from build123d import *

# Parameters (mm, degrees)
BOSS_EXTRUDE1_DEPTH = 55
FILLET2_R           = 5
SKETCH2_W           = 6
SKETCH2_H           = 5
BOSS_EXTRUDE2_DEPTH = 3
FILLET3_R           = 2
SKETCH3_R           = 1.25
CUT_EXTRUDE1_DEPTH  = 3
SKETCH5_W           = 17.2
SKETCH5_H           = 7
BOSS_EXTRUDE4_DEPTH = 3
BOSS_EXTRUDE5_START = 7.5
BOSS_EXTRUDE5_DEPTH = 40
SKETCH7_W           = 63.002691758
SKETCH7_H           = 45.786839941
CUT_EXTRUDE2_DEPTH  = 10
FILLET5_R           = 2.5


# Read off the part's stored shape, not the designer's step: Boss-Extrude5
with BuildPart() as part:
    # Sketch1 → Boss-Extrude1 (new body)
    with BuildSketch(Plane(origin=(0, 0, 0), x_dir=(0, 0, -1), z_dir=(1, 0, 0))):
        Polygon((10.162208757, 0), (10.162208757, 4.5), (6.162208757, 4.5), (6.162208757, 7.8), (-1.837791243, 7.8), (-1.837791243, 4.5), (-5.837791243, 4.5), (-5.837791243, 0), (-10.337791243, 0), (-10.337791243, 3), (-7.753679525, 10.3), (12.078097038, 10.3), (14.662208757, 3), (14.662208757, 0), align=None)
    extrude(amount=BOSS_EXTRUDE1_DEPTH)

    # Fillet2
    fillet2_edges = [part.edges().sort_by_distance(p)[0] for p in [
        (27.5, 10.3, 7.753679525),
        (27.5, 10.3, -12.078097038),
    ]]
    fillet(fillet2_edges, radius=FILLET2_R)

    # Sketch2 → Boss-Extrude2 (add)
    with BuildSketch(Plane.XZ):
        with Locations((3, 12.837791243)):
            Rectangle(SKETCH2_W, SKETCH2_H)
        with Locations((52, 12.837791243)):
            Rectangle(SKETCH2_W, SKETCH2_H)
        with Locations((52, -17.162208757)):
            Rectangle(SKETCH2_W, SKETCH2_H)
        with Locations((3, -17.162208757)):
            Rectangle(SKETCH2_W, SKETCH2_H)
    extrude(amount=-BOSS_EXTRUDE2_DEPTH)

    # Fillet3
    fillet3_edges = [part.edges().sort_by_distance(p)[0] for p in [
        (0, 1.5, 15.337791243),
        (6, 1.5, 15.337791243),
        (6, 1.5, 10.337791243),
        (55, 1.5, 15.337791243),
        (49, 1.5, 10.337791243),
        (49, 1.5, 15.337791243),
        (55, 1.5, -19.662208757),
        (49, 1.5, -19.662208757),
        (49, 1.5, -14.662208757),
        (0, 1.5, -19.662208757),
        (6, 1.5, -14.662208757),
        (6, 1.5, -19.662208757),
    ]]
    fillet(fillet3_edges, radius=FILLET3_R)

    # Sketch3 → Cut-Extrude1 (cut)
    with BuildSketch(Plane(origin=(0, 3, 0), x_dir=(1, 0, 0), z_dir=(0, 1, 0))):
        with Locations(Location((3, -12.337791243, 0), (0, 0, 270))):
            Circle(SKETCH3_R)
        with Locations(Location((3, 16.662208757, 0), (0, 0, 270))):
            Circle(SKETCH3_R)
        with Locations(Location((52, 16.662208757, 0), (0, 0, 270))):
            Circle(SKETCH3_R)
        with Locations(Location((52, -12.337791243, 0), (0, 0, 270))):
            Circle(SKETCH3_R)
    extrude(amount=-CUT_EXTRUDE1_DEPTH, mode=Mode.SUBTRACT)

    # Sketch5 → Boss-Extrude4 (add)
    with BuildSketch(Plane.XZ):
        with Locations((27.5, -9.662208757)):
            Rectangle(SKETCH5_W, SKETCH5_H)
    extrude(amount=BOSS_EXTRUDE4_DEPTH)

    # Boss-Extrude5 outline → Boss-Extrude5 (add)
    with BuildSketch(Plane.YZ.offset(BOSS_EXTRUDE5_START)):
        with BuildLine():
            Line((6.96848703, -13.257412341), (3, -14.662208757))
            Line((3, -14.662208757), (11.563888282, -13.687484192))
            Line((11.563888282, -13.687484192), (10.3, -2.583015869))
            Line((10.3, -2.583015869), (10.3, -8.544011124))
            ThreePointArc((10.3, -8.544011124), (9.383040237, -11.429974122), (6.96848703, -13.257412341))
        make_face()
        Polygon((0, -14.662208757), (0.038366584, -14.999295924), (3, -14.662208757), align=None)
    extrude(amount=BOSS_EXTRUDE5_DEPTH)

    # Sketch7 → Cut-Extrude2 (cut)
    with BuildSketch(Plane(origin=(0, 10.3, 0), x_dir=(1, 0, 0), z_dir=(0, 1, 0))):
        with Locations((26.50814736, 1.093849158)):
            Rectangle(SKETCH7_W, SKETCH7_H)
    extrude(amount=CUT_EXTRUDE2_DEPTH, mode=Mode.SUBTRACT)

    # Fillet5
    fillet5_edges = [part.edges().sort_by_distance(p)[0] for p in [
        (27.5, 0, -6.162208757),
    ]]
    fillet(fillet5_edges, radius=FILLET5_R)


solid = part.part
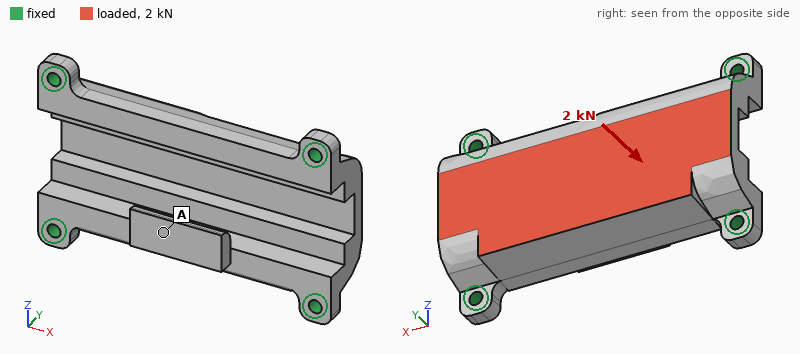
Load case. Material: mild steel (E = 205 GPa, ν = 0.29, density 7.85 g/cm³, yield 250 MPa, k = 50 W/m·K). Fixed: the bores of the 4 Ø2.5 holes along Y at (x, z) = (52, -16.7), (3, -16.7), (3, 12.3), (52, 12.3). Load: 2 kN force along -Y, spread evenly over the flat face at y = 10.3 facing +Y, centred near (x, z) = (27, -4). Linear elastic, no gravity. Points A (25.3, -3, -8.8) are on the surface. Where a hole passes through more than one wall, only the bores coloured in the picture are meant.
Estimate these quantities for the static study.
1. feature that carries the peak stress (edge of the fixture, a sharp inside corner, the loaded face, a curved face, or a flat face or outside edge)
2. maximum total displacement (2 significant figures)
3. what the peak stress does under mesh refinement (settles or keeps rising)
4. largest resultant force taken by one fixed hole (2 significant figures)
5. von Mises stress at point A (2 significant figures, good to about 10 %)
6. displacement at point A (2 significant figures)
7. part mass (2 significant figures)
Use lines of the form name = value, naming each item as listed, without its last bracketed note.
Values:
feature that carries the peak stress = edge of the fixture
maximum total displacement = 9.8 µm
what the peak stress does under mesh refinement = keeps rising
largest resultant force taken by one fixed hole = 850 N
von Mises stress at point A = 10.0 MPa
displacement at point A = 9.0 µm
part mass = 66 g
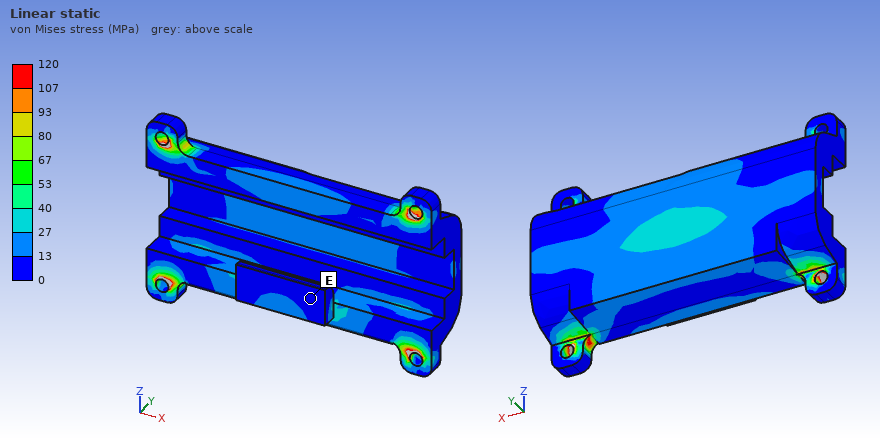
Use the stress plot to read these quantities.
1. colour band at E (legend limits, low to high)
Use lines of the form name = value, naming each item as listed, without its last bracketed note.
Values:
colour band at E = 0 to 13 MPa
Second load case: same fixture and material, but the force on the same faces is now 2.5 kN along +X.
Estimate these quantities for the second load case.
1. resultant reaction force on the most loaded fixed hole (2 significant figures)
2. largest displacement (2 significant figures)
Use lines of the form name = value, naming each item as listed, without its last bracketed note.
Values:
resultant reaction force on the most loaded fixed hole = 730 N
largest displacement = 4.4 µm
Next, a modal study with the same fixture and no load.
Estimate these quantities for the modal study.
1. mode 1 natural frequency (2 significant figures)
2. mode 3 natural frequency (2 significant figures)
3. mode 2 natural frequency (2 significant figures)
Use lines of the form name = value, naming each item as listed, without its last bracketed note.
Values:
mode 1 natural frequency = 10 kHz
mode 3 natural frequency = 16 kHz
mode 2 natural frequency = 11 kHz
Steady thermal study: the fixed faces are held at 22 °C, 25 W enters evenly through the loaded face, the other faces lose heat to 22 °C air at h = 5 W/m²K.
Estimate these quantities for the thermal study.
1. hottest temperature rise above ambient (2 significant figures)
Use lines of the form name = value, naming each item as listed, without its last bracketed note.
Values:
hottest temperature rise above ambient = 49 K
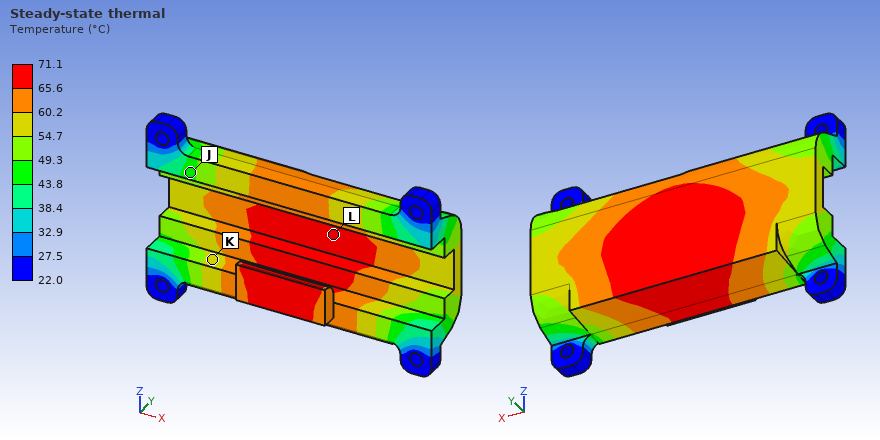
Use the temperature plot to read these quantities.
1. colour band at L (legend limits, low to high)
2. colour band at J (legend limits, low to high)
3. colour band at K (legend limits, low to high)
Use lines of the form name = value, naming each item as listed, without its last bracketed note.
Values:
colour band at L = 65.6 to 71.1 °C
colour band at J = 43.8 to 49.3 °C
colour band at K = 54.7 to 60.2 °C
